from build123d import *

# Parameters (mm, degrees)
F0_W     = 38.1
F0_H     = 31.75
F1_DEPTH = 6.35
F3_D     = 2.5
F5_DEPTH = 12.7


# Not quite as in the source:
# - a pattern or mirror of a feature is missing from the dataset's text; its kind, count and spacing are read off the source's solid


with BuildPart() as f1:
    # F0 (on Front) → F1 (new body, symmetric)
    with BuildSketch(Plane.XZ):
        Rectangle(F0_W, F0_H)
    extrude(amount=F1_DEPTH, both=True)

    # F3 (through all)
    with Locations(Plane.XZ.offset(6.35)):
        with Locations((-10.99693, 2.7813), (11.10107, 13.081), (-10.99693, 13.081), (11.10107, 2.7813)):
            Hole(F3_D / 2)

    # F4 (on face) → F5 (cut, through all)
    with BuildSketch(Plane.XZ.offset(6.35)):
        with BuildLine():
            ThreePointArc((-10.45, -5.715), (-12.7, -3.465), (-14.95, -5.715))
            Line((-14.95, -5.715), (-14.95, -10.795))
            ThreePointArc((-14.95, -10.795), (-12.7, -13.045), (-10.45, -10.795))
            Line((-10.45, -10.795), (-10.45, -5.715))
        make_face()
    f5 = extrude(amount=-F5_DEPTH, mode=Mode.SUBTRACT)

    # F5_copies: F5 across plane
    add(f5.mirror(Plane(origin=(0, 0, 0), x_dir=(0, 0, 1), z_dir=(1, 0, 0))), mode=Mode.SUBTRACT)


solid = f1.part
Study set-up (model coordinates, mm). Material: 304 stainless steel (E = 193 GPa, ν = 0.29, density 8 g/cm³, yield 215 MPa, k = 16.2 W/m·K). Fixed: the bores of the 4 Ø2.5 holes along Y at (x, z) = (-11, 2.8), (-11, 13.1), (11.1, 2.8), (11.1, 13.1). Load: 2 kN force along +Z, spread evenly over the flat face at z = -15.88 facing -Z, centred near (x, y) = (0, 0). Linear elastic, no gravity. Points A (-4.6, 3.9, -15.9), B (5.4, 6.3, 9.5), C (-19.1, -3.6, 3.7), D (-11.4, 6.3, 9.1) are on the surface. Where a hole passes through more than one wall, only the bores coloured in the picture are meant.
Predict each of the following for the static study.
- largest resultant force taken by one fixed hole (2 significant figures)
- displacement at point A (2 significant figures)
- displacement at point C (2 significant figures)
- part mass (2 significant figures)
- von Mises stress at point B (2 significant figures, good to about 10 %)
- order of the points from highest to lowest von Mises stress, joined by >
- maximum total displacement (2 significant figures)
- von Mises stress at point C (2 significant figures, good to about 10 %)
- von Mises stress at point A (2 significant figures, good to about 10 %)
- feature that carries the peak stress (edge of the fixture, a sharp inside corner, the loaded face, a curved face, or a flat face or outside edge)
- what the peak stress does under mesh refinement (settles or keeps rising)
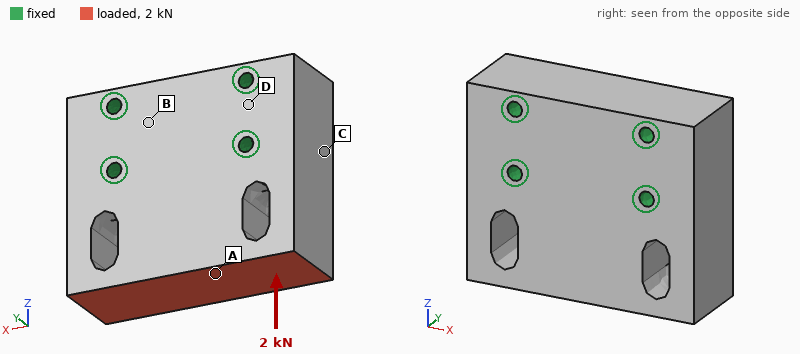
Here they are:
750 N
0.55 µm
0.19 µm
110 g
2.5 MPa
A > C > B > D
0.81 µm
4.0 MPa
5.6 MPa
edge of the fixture
keeps rising
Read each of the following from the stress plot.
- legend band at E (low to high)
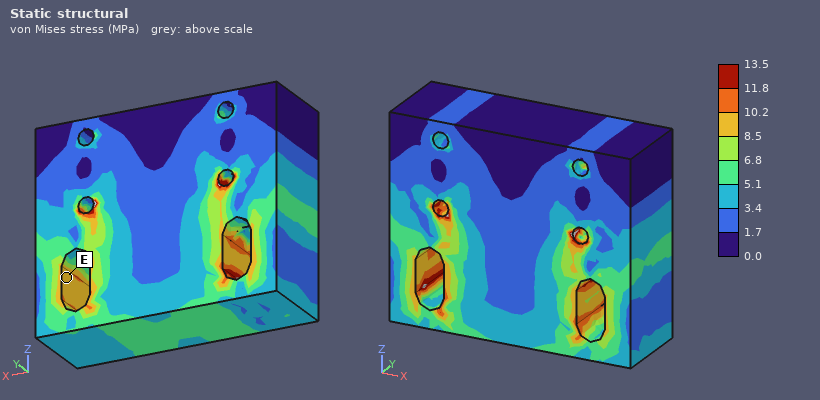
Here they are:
8.5 to 10.2 MPa
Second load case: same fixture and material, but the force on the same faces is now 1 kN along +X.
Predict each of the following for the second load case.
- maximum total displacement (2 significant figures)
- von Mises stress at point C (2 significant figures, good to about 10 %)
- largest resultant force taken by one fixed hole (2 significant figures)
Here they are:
1.5 µm
4.9 MPa
800 N
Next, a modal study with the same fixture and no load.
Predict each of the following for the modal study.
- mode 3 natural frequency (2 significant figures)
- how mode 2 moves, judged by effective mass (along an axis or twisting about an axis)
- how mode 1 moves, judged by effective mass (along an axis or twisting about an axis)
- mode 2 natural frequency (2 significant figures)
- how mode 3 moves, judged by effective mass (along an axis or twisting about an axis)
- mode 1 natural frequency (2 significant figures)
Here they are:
29 kHz
twisting about Z
along Y
26 kHz
along X
18 kHz
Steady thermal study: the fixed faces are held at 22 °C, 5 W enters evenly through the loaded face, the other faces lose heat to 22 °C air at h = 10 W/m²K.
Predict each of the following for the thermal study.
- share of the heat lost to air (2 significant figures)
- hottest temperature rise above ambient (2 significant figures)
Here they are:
4.2 %
16 K
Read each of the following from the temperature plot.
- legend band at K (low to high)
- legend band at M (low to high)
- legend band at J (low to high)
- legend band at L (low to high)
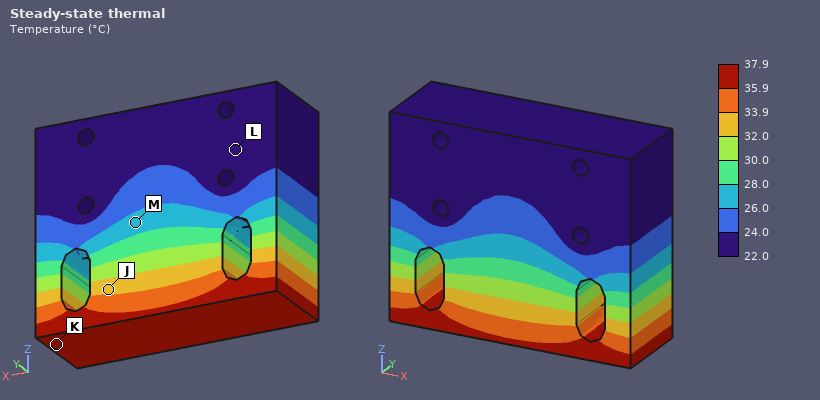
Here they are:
35.9 to 37.9 °C
26.0 to 28.0 °C
32.0 to 33.9 °C
22.0 to 24.0 °C
